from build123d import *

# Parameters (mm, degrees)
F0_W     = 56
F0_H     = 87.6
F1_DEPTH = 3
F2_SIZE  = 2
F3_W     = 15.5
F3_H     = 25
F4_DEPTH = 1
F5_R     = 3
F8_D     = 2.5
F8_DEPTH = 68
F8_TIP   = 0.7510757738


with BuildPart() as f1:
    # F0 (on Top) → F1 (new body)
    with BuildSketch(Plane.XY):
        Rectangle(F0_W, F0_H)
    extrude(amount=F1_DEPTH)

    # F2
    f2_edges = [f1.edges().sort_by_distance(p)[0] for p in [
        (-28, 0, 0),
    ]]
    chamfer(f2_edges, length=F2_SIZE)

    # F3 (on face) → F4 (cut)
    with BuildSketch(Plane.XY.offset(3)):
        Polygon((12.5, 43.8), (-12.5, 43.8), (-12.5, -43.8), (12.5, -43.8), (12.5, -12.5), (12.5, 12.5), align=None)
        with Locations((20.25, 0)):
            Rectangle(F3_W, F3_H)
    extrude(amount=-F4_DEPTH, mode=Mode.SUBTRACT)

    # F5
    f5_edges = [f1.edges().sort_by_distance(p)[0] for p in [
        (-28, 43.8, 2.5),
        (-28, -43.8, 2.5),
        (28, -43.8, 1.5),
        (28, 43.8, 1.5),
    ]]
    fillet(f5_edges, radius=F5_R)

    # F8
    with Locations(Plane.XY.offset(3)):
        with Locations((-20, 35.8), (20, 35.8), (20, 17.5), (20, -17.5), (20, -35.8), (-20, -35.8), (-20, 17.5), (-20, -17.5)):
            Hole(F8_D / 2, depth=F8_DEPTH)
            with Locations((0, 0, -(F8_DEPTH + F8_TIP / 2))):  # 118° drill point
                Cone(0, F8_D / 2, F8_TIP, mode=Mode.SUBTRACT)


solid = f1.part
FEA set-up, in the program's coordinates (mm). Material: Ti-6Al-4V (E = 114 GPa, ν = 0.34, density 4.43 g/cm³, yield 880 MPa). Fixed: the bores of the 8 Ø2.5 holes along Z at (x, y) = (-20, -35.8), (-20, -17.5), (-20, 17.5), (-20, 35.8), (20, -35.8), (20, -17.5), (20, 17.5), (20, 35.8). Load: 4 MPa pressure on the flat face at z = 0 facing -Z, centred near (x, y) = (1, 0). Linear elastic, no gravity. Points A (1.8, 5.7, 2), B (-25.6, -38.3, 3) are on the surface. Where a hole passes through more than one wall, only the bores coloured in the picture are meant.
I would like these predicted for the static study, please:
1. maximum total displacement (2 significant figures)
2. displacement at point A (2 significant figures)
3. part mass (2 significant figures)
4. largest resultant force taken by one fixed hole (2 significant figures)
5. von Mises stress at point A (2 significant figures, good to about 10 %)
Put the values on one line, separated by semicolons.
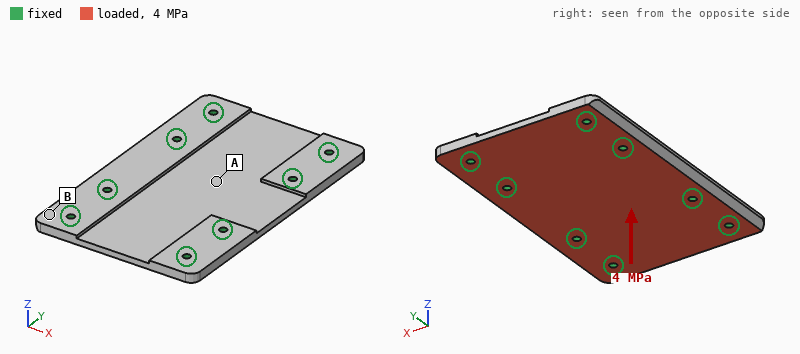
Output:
0.35 mm; 0.33 mm; 52 g; 3.6 kN; 260 MPa
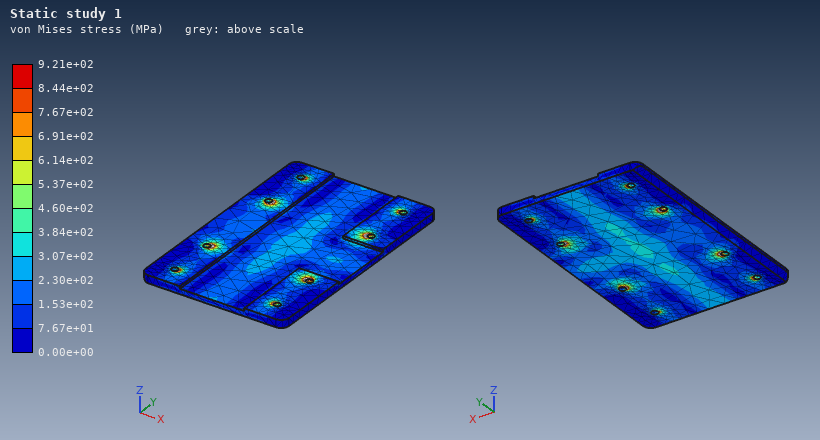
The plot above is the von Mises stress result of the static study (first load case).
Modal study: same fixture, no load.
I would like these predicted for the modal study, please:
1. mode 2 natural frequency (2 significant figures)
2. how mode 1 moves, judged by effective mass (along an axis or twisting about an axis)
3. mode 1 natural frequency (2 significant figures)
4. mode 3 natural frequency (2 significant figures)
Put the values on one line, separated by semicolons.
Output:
9100 Hz; along Z; 7000 Hz; 9300 Hz
